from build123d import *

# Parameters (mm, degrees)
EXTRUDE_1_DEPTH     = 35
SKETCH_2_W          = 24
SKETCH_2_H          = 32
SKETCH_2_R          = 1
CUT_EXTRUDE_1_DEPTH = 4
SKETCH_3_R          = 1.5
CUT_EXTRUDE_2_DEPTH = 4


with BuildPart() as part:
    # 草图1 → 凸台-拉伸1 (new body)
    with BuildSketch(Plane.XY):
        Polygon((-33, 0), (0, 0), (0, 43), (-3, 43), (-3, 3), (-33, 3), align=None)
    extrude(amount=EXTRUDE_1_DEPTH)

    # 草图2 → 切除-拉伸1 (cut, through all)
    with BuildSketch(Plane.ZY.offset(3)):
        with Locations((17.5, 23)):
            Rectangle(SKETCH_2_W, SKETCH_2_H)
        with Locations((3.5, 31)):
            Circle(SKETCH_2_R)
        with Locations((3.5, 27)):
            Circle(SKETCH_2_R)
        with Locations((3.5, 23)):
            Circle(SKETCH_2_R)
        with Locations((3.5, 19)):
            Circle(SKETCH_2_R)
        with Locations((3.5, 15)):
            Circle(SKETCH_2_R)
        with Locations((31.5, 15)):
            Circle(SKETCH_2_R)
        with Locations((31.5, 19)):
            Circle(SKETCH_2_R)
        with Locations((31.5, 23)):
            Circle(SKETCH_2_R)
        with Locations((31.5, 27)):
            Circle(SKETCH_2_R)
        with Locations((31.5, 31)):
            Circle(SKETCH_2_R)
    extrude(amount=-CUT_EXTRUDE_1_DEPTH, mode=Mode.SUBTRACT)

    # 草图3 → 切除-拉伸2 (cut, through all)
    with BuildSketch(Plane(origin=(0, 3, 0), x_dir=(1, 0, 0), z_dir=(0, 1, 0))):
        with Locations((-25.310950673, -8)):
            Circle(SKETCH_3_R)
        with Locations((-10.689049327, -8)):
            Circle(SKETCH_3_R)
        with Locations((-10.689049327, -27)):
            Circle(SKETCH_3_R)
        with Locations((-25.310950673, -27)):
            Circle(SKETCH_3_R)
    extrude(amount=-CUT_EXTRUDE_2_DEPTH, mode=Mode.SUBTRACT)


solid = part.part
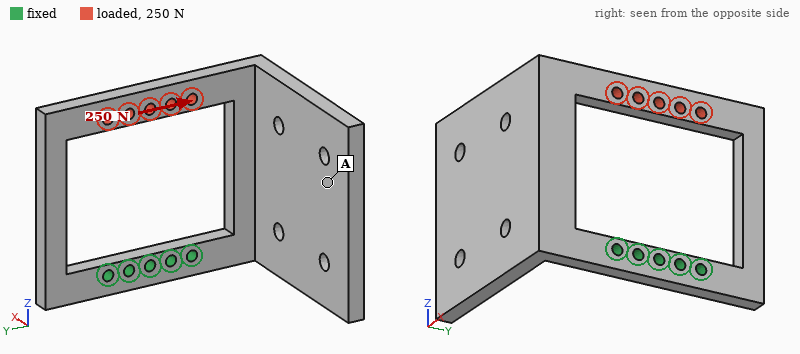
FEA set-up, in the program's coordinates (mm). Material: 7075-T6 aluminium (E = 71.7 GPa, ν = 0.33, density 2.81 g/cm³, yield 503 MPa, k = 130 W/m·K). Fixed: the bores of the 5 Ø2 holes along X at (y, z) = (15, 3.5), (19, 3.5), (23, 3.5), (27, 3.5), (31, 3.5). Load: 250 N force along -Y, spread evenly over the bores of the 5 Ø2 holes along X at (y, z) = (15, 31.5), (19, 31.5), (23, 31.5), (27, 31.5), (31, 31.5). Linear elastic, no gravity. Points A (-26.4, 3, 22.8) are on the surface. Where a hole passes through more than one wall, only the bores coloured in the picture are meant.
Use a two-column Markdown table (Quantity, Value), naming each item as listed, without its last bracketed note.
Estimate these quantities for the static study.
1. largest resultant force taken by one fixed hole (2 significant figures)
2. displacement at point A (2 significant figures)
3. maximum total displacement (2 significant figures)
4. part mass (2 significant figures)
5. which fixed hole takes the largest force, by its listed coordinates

| Quantity | Value |
|---|---|
| largest resultant force taken by one fixed hole | 540 N |
| displacement at point A | 0.23 mm |
| maximum total displacement | 0.37 mm |
| part mass | 15 g |
| which fixed hole takes the largest force, by its listed coordinates | (15, 3.5) |
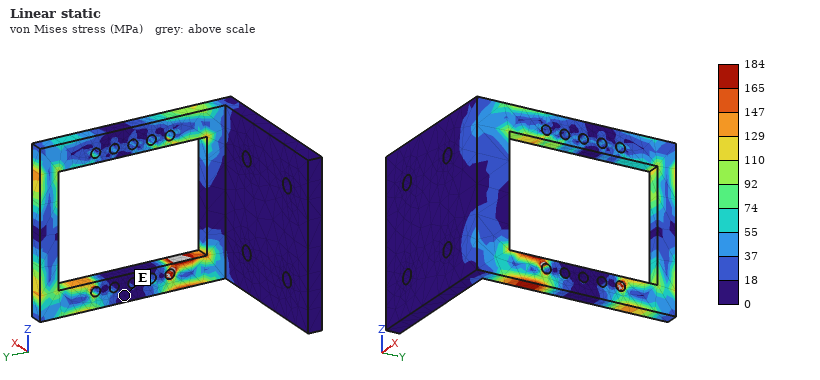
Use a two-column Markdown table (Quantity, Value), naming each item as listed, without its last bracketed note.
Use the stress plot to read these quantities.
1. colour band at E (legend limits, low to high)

| Quantity | Value |
|---|---|
| colour band at E | 0 to 18 MPa |
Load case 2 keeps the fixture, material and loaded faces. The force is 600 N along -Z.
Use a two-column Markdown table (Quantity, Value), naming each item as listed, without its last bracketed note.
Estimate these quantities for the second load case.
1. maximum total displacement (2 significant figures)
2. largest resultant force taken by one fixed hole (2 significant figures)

| Quantity | Value |
|---|---|
| maximum total displacement | 0.16 mm |
| largest resultant force taken by one fixed hole | 540 N |
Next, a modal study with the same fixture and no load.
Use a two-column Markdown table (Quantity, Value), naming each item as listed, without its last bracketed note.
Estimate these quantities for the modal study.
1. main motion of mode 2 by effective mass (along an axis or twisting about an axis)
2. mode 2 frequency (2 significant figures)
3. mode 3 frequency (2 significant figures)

| Quantity | Value |
|---|---|
| main motion of mode 2 by effective mass | along Y |
| mode 2 frequency | 830 Hz |
| mode 3 frequency | 1900 Hz |
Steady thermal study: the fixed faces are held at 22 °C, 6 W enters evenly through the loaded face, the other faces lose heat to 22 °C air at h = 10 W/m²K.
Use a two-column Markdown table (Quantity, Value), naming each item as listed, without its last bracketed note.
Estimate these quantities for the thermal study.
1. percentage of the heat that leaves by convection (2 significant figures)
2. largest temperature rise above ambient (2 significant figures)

| Quantity | Value |
|---|---|
| percentage of the heat that leaves by convection | 17 % |
| largest temperature rise above ambient | 57 K |
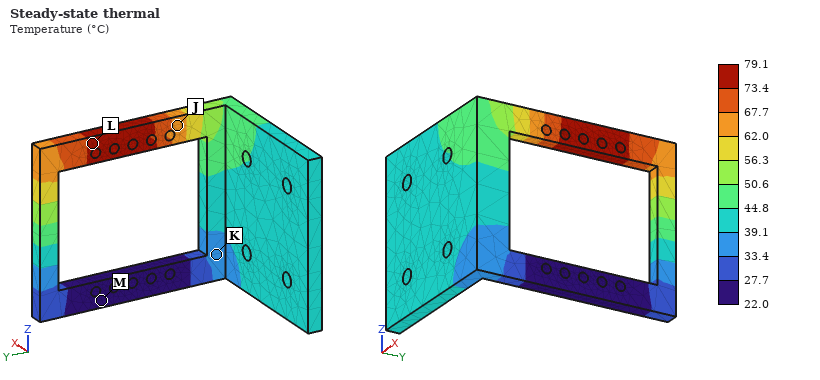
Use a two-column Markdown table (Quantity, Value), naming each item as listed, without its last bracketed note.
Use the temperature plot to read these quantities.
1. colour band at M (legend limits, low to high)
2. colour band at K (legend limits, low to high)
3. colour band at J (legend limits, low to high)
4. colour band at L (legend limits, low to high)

| Quantity | Value |
|---|---|
| colour band at M | 22.0 to 27.7 °C |
| colour band at K | 33.4 to 39.1 °C |
| colour band at J | 62.0 to 67.7 °C |
| colour band at L | 73.4 to 79.1 °C |
